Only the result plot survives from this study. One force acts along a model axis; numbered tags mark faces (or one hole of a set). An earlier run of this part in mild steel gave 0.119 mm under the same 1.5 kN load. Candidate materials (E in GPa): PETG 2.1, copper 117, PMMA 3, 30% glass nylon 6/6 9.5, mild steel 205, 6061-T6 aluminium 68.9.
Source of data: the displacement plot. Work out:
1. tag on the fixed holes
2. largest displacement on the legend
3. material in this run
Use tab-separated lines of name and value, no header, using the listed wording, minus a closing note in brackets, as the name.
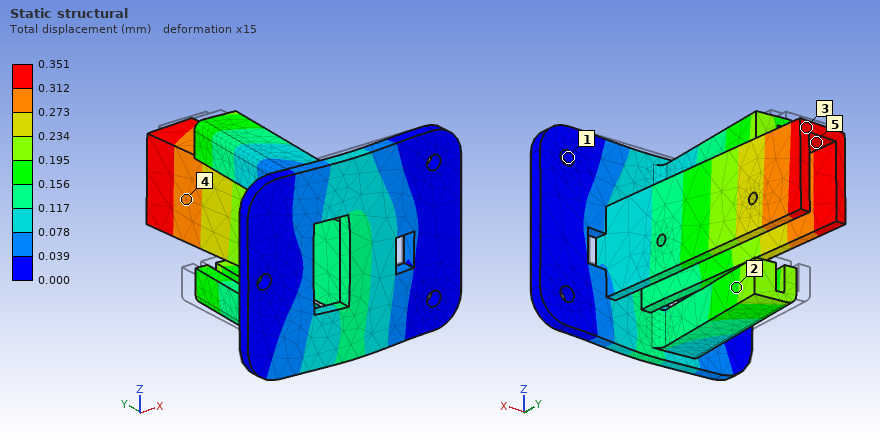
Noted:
tag on the fixed holes	1
largest displacement on the legend	0.351 mm
material in this run	6061-T6 aluminium
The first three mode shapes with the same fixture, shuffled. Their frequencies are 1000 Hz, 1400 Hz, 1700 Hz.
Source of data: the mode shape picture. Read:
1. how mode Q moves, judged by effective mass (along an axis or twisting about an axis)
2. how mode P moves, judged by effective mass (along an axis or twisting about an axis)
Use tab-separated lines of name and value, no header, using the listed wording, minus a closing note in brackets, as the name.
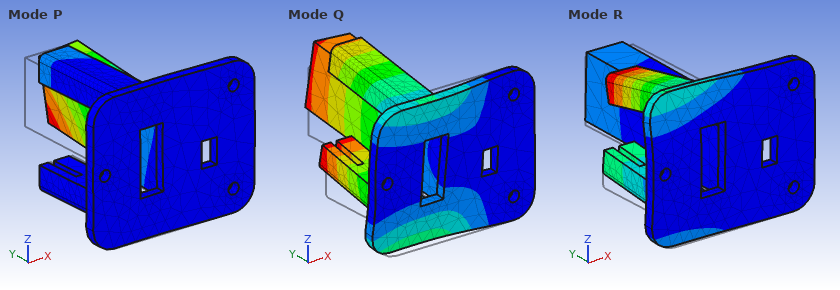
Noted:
how mode Q moves, judged by effective mass	along Z
how mode P moves, judged by effective mass	along X
